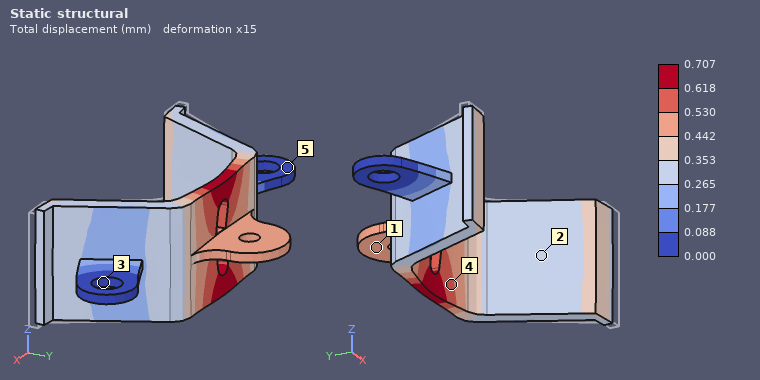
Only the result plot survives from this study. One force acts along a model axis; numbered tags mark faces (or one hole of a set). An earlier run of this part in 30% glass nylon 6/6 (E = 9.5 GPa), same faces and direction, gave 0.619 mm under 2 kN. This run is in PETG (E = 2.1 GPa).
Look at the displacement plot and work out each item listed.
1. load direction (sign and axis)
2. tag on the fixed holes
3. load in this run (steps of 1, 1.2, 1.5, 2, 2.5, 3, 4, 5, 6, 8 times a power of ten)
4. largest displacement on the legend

+Y
3
500 N
0.707 mm
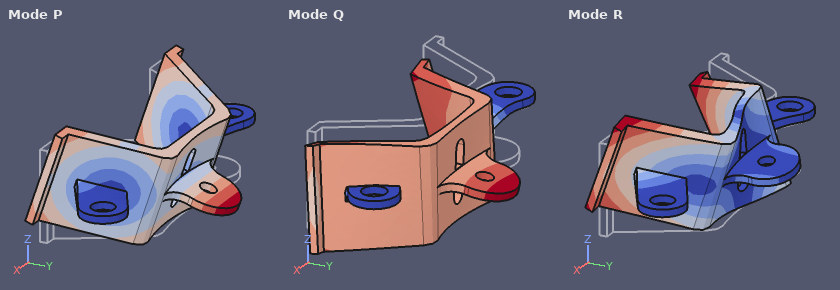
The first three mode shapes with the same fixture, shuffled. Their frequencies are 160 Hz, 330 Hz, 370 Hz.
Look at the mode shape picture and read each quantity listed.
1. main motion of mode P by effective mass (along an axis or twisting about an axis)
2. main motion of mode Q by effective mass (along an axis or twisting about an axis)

twisting about X
along Z
